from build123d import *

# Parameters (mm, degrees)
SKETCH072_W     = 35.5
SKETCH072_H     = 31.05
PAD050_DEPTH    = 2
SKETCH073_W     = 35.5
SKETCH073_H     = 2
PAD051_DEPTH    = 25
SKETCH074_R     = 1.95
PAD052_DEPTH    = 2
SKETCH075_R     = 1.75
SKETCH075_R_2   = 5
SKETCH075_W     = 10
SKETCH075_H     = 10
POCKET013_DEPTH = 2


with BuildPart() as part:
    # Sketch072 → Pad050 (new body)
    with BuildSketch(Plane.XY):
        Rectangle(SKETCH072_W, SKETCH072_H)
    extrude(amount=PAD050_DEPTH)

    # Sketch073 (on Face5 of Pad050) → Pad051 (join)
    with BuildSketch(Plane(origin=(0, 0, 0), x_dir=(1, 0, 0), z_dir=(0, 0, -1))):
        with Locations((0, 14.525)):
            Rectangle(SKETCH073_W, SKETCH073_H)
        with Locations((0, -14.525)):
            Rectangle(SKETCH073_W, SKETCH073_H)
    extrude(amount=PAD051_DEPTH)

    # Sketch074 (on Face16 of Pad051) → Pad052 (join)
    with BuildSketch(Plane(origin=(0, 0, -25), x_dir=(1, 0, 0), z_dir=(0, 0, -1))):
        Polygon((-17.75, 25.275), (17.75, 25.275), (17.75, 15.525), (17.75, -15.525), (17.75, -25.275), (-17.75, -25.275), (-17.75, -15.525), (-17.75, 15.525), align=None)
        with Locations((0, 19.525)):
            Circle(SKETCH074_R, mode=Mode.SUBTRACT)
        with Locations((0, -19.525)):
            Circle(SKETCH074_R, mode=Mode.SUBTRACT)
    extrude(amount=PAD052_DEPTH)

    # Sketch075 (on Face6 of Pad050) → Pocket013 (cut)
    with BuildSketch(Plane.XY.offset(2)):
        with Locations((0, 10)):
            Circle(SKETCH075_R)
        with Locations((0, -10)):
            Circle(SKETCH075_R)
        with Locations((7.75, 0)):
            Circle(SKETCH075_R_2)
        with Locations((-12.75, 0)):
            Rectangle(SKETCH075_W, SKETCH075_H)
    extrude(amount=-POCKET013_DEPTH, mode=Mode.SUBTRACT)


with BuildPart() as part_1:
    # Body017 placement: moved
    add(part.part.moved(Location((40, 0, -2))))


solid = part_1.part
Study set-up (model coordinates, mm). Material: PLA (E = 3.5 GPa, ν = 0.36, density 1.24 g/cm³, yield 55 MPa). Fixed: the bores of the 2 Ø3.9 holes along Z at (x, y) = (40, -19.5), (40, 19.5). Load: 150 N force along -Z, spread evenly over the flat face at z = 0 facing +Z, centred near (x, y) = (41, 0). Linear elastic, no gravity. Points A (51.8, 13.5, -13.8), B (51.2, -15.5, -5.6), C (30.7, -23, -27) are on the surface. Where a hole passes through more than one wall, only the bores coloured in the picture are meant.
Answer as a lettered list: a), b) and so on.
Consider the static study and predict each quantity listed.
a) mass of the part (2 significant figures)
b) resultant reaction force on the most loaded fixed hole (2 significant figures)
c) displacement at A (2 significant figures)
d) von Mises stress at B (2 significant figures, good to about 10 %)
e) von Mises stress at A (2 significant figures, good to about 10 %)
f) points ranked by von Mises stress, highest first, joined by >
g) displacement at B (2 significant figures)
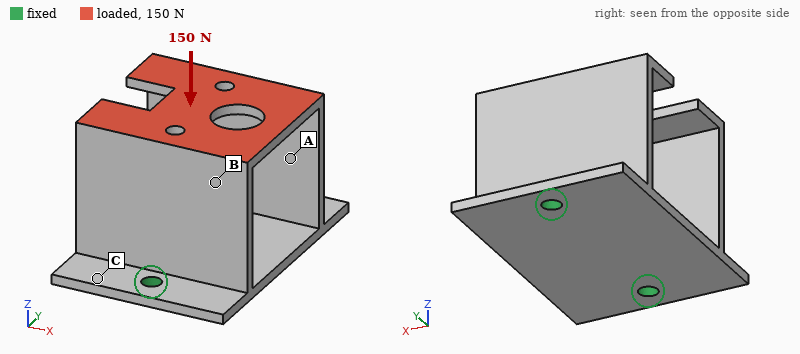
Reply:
a) 11 g
b) 76 N
c) 0.094 mm
d) 6.7 MPa
e) 3.7 MPa
f) B > A > C
g) 0.095 mm
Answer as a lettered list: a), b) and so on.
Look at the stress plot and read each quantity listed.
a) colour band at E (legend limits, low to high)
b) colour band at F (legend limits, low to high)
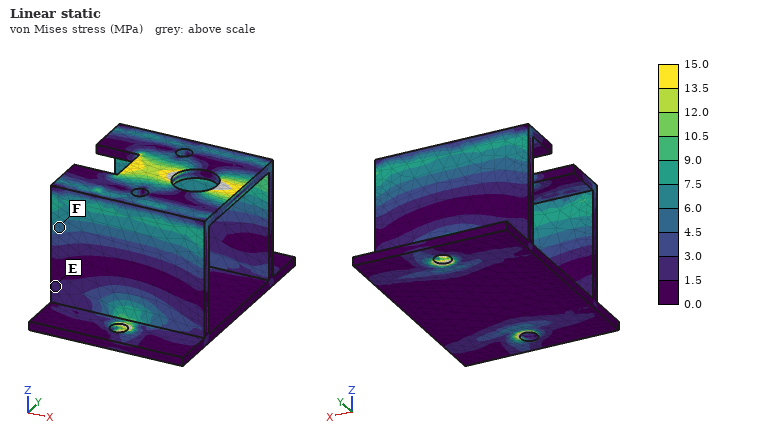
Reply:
a) 1.5 to 3.0 MPa
b) 4.5 to 6.0 MPa
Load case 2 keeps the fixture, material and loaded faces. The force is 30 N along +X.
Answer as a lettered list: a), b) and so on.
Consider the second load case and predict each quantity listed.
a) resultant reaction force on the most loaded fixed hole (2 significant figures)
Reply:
a) 15 N
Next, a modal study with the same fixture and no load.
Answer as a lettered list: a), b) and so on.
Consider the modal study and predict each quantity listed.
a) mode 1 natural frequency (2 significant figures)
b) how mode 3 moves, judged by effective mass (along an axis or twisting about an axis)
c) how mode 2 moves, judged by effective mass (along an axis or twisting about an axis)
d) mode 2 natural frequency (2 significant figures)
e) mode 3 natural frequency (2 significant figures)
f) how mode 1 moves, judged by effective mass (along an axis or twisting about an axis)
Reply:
a) 580 Hz
b) twisting about Z
c) along Y
d) 660 Hz
e) 1100 Hz
f) along X
